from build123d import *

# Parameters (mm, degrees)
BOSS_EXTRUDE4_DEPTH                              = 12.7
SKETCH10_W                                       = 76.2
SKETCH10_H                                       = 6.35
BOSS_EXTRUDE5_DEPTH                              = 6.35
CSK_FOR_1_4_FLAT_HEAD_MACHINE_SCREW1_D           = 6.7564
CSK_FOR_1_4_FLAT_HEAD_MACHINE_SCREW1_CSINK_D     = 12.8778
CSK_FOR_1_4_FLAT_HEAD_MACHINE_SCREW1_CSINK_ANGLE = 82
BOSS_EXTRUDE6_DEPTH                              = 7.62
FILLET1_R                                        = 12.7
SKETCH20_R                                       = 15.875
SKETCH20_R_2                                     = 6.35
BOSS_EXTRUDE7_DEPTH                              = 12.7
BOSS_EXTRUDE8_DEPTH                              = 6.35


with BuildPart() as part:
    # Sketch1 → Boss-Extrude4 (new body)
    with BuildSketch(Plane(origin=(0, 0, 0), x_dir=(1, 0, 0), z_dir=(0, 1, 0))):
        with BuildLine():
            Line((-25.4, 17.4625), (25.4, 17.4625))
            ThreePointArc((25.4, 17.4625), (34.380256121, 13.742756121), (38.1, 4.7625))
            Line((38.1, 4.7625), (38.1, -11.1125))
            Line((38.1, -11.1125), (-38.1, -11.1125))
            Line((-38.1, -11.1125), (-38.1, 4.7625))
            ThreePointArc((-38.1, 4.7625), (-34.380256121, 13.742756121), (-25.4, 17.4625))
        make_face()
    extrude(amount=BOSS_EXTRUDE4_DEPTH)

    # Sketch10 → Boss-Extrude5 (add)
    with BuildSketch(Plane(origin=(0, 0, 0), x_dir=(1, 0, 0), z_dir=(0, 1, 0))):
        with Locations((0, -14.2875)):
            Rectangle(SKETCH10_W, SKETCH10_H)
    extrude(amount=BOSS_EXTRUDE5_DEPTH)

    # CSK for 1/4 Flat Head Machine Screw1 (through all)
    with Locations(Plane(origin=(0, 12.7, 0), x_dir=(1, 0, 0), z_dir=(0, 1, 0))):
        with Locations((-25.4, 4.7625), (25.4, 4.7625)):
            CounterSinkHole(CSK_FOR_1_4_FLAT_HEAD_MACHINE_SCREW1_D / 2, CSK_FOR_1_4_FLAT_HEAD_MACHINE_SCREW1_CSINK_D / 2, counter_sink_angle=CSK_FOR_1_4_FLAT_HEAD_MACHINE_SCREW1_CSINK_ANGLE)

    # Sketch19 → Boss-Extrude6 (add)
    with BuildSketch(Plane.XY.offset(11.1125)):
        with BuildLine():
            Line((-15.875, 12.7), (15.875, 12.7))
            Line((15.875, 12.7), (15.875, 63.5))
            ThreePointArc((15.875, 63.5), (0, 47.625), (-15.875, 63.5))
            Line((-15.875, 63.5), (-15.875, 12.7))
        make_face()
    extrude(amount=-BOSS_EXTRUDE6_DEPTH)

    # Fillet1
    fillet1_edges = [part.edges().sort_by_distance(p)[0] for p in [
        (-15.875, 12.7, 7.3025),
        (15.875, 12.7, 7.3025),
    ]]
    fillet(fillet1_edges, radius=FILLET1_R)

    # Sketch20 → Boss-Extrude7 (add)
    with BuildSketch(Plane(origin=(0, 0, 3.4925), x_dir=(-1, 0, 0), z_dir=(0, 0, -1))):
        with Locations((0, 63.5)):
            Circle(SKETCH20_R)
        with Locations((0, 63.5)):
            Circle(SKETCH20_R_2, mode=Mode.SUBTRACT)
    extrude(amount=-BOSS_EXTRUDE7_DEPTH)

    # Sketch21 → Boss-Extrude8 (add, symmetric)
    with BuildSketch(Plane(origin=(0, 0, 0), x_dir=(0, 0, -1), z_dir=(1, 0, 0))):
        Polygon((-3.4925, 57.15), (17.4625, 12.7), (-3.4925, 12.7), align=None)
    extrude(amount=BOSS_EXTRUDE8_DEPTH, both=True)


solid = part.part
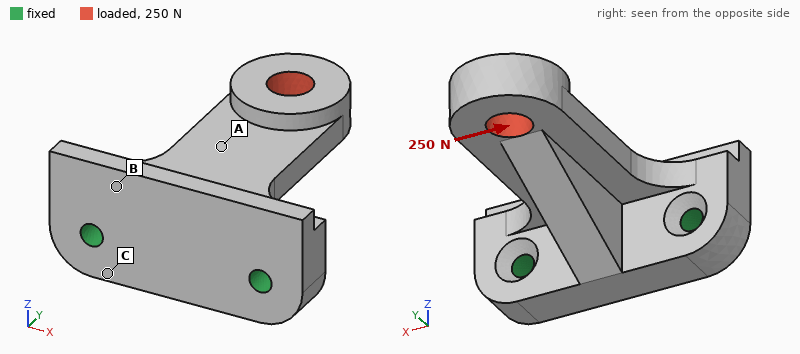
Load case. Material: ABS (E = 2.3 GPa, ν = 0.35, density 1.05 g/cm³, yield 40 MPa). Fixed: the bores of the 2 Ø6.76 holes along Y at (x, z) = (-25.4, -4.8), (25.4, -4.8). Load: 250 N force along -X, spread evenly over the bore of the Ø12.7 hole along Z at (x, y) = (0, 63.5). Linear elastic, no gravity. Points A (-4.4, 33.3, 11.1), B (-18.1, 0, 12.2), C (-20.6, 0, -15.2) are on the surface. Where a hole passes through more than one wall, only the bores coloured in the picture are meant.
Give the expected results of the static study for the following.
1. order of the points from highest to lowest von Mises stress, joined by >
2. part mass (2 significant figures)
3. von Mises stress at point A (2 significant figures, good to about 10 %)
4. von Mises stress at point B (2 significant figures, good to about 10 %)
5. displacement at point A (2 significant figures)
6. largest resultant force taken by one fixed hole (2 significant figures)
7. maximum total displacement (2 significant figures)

A > B > C
55 g
3.9 MPa
1.9 MPa
0.11 mm
340 N
0.51 mm
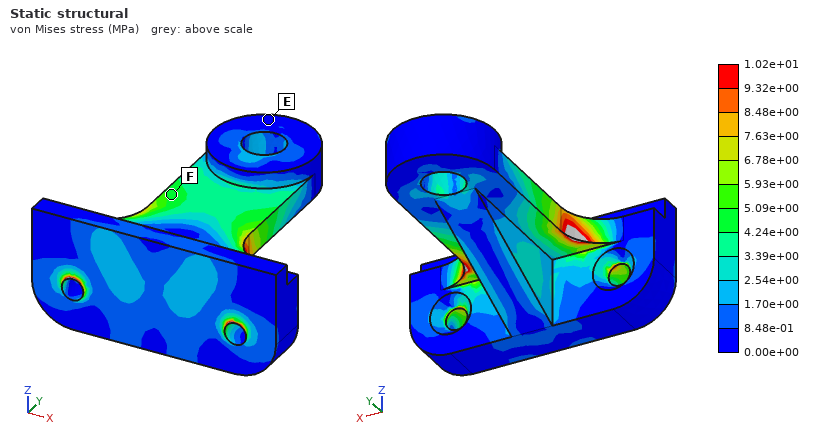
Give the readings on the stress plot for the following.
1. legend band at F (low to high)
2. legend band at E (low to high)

4.24e+00 to 5.09e+00 MPa
0.00e+00 to 8.48e-01 MPa
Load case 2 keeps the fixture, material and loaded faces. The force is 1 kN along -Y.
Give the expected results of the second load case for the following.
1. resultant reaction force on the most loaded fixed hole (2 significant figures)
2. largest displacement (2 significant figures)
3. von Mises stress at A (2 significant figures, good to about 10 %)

530 N
1.3 mm
6.8 MPa
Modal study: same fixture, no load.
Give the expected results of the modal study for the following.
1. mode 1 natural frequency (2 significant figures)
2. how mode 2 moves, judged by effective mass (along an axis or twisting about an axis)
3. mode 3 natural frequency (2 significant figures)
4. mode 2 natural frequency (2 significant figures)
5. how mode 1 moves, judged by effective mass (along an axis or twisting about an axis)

670 Hz
along X
2300 Hz
1200 Hz
along Z
